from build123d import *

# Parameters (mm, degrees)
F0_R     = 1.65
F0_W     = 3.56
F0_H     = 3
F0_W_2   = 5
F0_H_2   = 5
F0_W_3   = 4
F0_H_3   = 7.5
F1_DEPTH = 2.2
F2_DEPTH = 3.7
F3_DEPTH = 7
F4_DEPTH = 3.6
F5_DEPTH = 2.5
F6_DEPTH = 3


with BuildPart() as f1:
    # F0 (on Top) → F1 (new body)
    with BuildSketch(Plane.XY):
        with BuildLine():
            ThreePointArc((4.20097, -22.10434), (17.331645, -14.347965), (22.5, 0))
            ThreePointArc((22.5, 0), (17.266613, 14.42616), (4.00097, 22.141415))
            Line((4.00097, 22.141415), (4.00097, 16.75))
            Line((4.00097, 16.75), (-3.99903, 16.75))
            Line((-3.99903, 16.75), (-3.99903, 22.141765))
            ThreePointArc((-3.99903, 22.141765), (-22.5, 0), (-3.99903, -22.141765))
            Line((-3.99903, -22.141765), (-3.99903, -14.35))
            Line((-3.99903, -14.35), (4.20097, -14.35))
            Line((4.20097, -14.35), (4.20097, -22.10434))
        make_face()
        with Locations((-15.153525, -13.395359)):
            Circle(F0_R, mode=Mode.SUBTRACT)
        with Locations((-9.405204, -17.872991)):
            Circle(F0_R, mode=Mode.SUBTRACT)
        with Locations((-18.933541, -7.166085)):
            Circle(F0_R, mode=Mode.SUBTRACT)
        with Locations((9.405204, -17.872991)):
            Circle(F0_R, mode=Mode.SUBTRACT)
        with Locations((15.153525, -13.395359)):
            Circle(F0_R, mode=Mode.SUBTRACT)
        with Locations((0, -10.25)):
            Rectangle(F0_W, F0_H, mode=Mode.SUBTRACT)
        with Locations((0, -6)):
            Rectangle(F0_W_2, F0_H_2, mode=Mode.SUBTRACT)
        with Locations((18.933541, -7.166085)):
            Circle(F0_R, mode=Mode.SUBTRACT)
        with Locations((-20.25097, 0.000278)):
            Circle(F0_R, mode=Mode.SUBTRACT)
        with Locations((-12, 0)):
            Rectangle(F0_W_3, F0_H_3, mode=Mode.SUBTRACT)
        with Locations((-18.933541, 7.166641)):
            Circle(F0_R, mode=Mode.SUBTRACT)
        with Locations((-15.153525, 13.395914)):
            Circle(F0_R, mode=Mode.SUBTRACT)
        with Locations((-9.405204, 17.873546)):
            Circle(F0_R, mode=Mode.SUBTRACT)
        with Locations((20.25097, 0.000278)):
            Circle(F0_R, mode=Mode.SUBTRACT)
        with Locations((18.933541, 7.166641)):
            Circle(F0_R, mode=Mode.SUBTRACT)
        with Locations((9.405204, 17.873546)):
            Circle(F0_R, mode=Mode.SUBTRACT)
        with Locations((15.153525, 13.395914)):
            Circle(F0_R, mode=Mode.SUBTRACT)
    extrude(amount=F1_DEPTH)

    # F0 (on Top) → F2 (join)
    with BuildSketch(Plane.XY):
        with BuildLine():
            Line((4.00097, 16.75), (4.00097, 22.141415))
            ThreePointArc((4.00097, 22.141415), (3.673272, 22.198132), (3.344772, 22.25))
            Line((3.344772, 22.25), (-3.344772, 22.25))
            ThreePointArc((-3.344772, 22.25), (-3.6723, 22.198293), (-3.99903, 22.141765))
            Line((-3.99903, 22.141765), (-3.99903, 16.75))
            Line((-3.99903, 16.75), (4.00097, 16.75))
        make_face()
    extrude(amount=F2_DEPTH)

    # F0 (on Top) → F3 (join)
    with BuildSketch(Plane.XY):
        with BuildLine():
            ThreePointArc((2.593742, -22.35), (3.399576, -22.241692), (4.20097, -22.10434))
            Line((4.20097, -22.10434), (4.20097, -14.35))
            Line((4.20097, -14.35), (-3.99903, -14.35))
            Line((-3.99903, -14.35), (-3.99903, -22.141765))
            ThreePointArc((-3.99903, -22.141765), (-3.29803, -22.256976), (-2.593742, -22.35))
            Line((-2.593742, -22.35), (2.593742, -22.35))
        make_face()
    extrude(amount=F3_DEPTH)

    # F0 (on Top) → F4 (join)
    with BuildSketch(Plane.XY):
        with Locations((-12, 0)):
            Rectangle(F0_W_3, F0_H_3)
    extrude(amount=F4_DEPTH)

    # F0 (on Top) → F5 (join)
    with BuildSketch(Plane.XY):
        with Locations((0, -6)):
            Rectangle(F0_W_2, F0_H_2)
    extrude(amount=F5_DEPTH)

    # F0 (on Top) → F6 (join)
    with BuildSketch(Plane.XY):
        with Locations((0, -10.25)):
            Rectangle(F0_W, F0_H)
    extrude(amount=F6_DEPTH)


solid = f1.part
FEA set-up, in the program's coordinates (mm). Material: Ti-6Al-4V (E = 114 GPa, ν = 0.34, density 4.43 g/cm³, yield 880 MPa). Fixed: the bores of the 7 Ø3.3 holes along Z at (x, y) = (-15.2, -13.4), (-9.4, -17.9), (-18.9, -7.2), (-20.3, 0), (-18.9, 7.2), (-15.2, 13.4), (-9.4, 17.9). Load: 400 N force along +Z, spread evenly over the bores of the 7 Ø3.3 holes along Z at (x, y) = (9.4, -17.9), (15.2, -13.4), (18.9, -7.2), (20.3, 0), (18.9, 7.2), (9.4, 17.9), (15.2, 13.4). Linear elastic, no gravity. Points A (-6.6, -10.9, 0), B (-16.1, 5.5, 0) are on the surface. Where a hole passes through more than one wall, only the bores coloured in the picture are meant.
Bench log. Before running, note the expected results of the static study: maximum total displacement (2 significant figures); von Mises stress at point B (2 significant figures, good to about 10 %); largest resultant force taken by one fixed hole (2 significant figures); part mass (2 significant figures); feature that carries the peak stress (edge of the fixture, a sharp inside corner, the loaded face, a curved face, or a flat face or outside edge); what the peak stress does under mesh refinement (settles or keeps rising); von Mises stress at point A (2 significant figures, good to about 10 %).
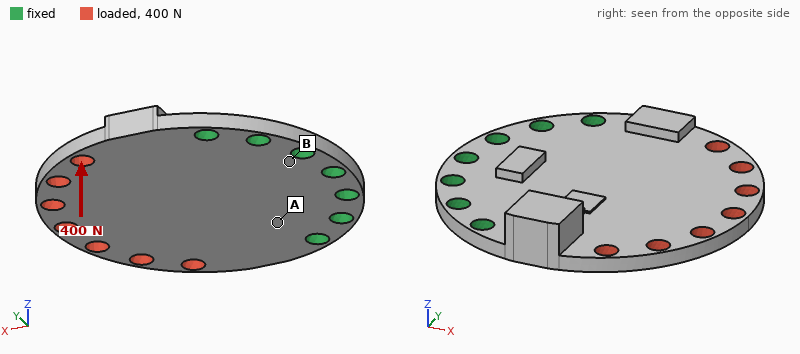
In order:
0.68 mm
75 MPa
370 N
16 g
edge of the fixture
keeps rising
190 MPa
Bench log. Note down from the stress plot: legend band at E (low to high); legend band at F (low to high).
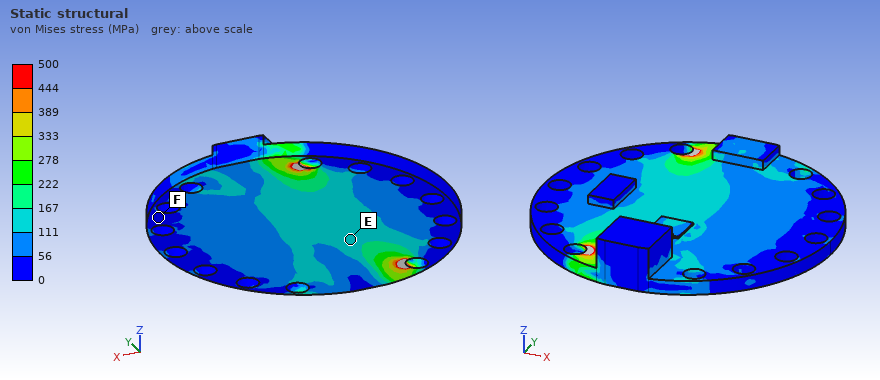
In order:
111 to 167 MPa
0 to 56 MPa
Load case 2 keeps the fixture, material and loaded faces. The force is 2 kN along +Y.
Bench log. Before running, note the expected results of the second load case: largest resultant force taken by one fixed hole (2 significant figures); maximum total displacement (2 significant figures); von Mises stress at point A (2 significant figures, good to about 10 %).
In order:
1.4 kN
27 µm
45 MPa
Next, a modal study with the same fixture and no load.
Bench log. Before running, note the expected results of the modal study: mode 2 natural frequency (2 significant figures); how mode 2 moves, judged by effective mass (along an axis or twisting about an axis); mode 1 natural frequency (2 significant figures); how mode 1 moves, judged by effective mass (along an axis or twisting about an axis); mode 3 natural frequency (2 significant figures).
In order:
5400 Hz
twisting about X
2300 Hz
along Z
9700 Hz
